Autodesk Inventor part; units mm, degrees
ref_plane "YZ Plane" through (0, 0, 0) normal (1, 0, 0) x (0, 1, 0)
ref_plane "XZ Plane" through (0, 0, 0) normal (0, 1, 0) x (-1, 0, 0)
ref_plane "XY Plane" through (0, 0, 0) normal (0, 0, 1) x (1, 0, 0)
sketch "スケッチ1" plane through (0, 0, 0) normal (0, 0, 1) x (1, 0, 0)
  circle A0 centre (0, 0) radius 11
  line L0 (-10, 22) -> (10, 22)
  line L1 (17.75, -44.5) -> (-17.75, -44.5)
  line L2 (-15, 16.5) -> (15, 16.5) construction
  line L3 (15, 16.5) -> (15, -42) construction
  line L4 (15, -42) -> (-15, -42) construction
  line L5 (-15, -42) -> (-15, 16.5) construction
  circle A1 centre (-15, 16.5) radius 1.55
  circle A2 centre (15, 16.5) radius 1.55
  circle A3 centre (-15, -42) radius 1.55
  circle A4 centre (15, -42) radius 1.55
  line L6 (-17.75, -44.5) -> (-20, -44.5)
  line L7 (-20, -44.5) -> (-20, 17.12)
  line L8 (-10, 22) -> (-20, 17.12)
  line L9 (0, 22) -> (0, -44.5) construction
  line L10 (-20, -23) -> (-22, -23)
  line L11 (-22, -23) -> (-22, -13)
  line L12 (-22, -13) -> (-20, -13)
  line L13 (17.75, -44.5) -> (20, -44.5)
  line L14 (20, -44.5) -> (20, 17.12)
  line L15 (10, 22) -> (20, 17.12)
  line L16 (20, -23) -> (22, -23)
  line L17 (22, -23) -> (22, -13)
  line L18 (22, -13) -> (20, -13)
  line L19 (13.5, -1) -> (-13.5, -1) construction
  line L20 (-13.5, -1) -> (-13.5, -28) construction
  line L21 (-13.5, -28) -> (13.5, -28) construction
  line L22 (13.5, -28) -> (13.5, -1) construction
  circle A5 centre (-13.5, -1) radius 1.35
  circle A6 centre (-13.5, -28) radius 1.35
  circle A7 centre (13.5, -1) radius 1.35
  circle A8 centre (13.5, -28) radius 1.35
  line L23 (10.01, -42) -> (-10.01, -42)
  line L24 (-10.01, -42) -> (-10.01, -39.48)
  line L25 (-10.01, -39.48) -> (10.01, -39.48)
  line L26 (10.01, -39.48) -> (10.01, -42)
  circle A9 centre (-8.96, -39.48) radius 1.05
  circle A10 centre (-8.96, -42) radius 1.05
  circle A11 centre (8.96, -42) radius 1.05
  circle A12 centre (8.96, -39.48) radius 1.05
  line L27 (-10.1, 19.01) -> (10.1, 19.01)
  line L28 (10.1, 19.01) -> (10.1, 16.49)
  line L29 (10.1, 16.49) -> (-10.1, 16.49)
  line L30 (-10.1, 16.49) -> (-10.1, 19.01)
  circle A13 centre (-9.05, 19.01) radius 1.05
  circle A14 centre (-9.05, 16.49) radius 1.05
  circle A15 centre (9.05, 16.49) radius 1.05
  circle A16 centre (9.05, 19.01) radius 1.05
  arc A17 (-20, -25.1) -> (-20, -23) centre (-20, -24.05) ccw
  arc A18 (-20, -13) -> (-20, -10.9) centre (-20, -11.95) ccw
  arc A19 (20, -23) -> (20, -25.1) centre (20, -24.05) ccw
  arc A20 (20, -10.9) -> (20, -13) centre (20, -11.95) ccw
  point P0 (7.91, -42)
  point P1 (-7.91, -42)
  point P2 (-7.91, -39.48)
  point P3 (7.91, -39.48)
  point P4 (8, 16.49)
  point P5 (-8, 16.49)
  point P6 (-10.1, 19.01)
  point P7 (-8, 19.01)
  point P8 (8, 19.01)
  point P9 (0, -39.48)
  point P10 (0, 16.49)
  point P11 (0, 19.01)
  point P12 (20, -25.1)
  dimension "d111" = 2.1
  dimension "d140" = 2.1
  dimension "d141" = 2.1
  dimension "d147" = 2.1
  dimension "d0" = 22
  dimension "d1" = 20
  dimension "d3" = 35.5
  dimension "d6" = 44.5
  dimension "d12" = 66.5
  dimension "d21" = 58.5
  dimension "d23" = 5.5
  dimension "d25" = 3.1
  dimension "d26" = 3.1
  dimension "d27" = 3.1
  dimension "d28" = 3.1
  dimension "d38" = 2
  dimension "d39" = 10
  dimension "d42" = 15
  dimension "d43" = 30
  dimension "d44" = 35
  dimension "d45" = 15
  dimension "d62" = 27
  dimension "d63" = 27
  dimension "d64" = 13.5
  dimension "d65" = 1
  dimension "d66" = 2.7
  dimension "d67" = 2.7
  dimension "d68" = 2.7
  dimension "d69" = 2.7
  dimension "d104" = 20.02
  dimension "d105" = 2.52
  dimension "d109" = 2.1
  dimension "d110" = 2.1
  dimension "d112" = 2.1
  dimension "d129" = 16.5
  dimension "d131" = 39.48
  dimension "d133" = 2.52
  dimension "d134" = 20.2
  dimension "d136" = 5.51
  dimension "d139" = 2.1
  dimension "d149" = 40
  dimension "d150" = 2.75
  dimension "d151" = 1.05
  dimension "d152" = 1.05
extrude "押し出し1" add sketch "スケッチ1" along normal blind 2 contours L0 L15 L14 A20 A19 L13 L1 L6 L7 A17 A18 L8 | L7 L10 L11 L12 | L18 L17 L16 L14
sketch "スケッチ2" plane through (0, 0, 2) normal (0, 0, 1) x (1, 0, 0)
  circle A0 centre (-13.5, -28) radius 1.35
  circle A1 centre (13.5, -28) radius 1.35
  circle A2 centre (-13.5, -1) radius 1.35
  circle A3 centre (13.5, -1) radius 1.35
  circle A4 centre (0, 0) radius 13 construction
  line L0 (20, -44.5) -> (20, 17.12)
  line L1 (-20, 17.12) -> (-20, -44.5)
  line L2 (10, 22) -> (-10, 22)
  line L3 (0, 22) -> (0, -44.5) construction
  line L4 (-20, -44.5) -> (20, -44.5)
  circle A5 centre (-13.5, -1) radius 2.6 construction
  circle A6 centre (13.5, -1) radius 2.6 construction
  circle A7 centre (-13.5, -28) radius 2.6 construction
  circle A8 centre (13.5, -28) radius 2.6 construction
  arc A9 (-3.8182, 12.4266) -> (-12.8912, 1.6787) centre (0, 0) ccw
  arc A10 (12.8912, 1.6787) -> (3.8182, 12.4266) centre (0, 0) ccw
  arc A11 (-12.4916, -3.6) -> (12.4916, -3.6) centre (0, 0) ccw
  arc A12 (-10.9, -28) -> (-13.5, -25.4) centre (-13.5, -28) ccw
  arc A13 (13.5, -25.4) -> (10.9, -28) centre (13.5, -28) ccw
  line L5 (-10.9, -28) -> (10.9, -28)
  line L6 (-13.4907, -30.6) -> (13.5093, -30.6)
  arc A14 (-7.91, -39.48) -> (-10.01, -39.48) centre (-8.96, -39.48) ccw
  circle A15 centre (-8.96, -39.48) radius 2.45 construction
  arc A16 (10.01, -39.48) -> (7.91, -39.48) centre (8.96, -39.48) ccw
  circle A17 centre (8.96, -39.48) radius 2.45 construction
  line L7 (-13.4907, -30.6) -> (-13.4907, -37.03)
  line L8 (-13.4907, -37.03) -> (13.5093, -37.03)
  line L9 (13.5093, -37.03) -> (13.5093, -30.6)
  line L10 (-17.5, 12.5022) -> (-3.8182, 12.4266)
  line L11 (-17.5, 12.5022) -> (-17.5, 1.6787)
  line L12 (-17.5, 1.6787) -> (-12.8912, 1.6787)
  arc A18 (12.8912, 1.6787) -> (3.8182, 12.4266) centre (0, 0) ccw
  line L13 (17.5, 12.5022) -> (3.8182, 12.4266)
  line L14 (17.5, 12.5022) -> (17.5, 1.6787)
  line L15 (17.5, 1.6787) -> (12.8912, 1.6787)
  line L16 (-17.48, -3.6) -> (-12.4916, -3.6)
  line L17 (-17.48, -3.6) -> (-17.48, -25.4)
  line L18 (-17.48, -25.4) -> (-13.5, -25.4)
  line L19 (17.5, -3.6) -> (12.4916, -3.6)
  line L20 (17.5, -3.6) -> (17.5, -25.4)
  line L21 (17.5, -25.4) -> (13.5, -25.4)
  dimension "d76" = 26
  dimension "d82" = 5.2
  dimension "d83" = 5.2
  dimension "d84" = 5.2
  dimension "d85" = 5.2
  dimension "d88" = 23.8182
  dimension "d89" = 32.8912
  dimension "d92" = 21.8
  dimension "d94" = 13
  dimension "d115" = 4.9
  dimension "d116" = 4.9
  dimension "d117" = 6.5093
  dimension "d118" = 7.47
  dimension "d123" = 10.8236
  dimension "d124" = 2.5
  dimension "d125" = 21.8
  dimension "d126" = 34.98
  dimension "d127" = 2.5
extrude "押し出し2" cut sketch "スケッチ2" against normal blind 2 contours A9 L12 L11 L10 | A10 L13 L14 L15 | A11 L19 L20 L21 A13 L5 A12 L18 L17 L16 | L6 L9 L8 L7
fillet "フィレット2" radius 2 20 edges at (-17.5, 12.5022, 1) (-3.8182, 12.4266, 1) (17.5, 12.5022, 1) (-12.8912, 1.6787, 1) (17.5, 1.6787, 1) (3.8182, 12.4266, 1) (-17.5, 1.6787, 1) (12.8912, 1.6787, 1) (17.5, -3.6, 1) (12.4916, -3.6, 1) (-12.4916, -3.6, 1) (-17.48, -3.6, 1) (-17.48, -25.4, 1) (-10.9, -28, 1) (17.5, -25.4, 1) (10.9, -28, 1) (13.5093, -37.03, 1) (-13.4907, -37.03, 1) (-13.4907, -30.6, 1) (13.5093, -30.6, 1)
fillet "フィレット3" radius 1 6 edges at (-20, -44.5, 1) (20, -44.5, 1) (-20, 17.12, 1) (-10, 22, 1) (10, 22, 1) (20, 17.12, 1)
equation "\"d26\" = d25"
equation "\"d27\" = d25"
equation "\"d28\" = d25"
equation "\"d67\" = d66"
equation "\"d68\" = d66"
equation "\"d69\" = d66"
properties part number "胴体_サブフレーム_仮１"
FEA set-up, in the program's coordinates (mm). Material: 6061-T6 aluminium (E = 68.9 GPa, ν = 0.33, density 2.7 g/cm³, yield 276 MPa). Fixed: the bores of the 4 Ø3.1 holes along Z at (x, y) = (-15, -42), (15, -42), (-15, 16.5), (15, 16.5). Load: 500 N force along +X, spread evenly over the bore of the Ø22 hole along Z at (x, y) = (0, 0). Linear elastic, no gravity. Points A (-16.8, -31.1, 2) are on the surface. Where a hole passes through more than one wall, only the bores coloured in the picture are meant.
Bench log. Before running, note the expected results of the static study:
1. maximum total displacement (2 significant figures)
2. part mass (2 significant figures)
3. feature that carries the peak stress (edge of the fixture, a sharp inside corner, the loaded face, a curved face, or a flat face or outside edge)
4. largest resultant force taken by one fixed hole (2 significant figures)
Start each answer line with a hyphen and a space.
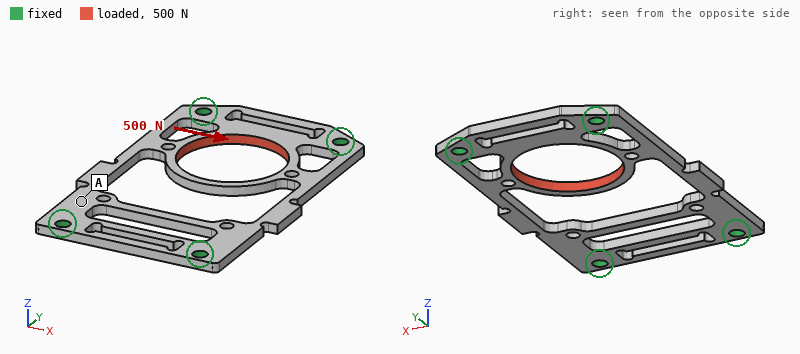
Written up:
- 89 µm
- 6.2 g
- a curved face
- 260 N
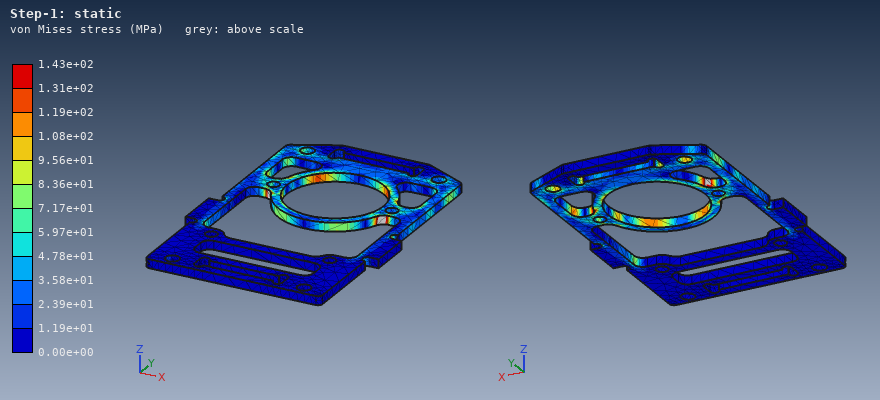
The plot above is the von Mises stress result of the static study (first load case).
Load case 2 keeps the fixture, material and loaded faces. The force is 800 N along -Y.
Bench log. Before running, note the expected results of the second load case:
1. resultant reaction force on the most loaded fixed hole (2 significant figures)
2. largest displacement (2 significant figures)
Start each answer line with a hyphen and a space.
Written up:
- 350 N
- 72 µm
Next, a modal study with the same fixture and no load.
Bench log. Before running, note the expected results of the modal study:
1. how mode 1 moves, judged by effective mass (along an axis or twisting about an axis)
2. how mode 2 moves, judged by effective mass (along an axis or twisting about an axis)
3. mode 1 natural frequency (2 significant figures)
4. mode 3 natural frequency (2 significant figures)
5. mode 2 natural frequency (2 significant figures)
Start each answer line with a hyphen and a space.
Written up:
- along Z
- twisting about Y
- 2600 Hz
- 4700 Hz
- 3500 Hz
